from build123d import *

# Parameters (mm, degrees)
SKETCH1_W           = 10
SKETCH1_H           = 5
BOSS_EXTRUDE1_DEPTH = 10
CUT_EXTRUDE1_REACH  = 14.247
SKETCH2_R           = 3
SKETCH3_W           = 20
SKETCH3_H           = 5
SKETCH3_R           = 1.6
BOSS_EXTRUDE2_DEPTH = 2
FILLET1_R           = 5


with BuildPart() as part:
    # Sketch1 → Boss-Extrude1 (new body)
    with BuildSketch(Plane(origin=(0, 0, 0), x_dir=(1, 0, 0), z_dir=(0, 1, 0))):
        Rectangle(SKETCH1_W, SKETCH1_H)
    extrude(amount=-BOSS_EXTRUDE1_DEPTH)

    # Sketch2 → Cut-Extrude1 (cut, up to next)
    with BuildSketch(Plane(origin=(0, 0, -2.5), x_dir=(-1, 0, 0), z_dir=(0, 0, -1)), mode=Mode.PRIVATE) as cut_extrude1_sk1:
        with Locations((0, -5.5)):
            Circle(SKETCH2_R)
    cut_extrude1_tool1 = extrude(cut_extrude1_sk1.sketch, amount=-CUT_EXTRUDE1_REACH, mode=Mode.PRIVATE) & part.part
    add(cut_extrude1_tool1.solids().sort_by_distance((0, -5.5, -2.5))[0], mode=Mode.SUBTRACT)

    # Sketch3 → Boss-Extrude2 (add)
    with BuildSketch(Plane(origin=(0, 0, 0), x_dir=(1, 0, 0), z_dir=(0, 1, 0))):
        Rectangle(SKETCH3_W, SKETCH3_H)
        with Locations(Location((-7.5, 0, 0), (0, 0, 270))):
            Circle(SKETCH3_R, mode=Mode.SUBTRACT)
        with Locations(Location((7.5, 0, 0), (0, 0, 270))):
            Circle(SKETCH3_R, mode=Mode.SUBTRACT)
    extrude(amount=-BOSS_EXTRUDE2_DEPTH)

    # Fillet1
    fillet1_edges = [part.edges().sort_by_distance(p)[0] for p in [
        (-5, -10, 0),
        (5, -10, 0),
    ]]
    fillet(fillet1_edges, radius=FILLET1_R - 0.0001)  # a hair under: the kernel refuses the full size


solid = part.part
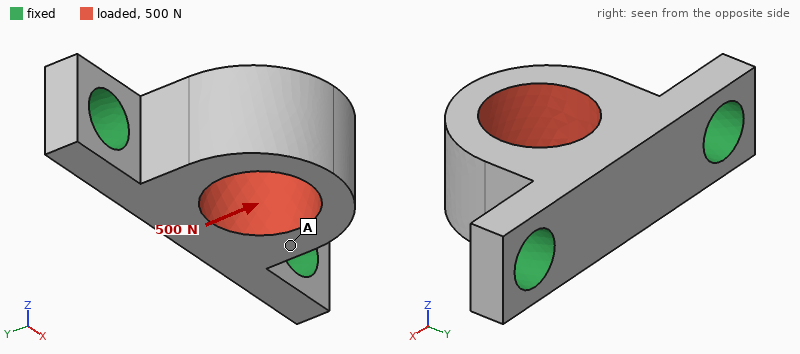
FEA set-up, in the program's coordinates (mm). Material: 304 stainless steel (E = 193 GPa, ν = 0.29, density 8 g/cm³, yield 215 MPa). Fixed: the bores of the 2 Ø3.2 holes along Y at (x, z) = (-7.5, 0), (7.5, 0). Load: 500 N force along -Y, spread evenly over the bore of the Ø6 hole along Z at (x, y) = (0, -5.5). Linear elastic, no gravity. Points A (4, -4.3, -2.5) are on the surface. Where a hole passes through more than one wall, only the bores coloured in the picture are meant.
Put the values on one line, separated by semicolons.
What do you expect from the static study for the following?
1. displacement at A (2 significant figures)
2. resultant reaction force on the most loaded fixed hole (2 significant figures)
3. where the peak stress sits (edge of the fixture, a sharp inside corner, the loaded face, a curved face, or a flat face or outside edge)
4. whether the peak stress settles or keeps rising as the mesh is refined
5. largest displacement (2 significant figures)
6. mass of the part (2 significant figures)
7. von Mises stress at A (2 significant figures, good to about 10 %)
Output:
1.6 µm; 270 N; edge of the fixture; keeps rising; 2.2 µm; 3.0 g; 22 MPa
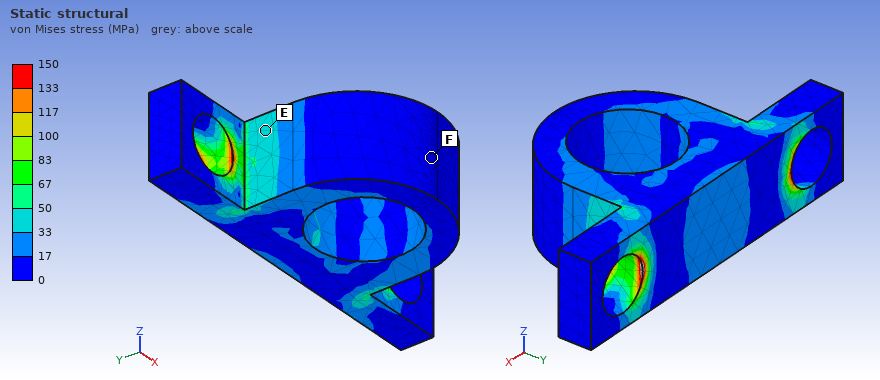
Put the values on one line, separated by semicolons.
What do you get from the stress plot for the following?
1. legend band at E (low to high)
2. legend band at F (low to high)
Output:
33 to 50 MPa; 0 to 17 MPa
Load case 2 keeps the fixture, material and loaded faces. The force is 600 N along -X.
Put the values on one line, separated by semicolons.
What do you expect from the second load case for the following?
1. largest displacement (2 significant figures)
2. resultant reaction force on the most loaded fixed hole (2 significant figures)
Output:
7.3 µm; 380 N
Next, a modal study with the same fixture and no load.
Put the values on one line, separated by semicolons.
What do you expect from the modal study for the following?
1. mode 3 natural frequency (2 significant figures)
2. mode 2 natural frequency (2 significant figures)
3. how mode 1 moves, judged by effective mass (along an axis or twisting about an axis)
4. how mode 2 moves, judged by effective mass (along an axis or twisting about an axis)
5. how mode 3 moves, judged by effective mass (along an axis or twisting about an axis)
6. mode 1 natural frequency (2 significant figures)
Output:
53 kHz; 40 kHz; along Z; along X; along Y; 21 kHz
